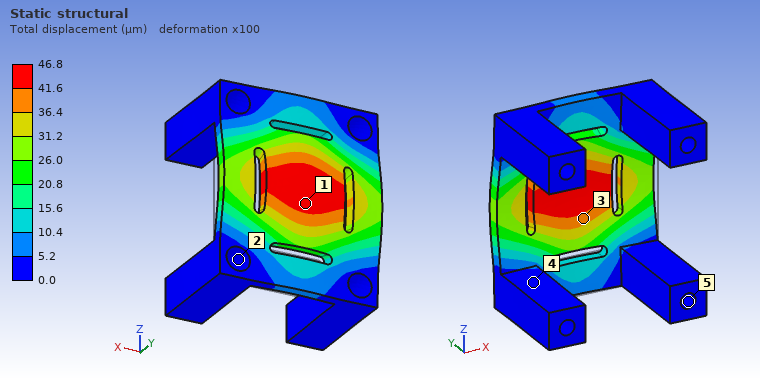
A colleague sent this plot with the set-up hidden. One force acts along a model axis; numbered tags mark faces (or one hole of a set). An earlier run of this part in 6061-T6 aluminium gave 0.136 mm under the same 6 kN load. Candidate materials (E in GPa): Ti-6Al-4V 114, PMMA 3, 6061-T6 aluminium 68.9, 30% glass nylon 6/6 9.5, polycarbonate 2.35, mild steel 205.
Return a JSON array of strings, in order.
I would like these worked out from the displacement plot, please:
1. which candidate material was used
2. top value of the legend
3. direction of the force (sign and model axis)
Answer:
["mild steel", "46.8 µm", "+Y"]
